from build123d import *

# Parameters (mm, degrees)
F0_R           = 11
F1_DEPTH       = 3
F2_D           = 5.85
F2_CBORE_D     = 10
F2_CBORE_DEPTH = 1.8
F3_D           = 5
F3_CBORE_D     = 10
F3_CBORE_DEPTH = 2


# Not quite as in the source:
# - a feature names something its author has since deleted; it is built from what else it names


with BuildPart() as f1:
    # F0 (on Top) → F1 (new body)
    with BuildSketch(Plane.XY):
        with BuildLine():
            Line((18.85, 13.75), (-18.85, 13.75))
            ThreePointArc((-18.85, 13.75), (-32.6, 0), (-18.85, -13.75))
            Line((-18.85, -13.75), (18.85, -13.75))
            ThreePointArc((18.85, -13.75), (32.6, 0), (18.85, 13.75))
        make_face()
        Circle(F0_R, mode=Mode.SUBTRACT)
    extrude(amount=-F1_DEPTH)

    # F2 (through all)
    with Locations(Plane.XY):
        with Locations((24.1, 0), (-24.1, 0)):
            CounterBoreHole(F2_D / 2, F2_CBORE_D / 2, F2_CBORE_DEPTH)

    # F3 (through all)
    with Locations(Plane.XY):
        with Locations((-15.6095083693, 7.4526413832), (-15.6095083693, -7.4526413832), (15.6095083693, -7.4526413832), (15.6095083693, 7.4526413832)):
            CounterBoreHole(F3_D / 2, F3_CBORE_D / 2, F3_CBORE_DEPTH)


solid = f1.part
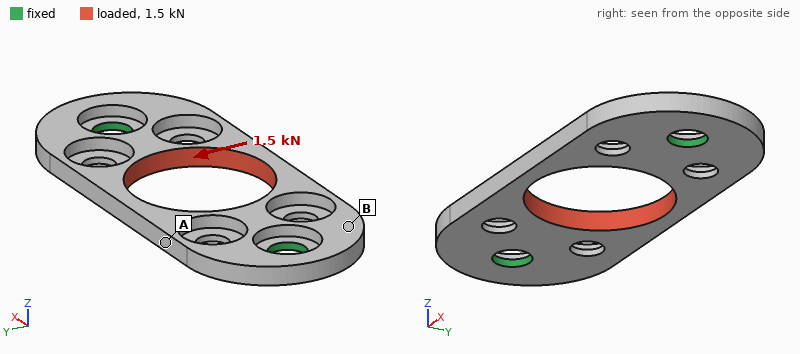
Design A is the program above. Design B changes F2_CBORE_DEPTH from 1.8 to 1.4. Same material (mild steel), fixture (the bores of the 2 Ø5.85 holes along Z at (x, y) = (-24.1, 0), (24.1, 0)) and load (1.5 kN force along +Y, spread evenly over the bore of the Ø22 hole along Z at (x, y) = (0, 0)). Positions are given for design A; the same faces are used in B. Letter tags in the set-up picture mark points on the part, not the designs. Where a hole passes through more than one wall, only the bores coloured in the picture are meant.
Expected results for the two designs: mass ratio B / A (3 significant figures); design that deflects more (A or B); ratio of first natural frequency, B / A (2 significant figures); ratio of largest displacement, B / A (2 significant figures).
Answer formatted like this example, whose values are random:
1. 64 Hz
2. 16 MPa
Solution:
1. 1.02
2. A
3. 1.1
4. 0.82
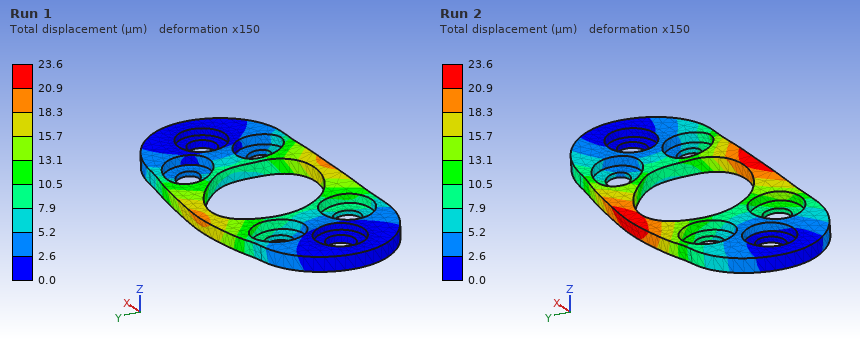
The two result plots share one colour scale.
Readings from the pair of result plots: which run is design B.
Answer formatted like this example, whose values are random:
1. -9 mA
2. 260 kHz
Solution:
1. Run 1
